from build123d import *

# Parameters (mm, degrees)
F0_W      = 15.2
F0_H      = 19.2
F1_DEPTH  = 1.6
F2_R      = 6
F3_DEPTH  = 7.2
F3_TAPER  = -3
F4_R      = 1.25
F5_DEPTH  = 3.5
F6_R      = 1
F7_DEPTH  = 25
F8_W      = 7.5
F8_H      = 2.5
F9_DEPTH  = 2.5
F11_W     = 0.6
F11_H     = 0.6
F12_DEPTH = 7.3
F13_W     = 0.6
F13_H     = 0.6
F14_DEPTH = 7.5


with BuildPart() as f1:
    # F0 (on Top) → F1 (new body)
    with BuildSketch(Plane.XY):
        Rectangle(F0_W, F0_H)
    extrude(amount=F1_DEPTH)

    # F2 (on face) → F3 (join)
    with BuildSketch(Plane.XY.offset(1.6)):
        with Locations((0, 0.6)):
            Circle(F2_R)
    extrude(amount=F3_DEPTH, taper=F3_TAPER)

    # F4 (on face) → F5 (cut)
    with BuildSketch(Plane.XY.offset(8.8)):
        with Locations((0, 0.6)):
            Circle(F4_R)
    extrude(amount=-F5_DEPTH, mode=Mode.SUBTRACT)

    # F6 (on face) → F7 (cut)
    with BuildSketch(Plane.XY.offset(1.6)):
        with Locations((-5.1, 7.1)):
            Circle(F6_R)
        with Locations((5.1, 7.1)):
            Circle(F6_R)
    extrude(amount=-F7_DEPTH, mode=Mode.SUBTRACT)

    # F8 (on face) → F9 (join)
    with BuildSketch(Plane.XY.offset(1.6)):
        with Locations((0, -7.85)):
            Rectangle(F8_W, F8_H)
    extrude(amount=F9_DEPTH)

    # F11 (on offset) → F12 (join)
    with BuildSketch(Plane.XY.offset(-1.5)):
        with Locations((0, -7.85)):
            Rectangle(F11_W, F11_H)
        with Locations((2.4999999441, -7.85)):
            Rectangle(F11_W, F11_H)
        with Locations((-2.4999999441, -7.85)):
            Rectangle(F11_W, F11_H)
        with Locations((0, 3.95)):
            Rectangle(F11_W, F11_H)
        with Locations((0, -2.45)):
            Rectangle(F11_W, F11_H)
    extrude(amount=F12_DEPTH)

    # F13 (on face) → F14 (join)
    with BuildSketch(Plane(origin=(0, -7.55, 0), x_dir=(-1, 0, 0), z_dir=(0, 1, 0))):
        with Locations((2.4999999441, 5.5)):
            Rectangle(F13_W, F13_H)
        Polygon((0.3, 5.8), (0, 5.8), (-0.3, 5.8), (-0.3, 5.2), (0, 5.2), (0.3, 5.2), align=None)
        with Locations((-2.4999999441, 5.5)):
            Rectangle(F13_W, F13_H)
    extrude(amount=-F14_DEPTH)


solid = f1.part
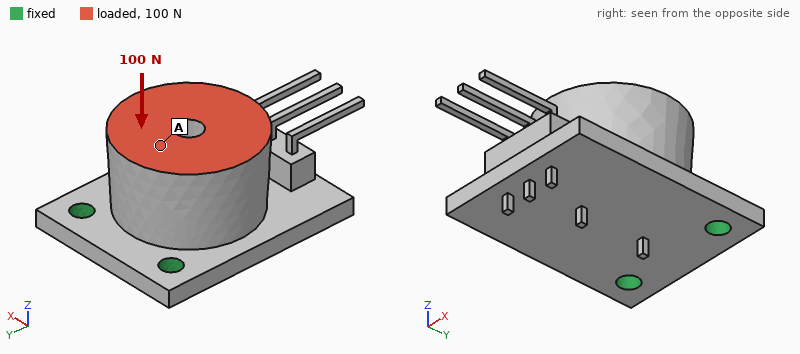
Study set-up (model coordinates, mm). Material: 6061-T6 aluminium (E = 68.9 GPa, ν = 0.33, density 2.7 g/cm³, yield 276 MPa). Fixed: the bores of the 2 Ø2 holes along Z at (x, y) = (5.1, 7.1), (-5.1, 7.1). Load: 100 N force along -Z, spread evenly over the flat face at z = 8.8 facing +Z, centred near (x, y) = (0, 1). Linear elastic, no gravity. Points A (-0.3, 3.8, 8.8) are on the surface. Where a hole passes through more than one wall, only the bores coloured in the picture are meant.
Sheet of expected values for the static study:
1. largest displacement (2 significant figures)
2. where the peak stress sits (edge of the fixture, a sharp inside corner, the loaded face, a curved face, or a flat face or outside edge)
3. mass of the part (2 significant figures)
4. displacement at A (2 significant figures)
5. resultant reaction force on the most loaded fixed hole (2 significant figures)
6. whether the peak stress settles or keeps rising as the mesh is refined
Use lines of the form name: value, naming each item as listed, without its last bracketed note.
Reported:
largest displacement: 66 µm
where the peak stress sits: edge of the fixture
mass of the part: 3.7 g
displacement at A: 25 µm
resultant reaction force on the most loaded fixed hole: 50 N
whether the peak stress settles or keeps rising as the mesh is refined: keeps rising
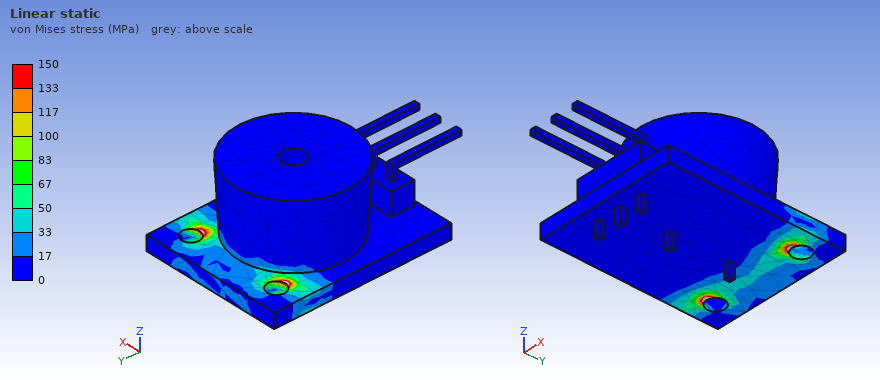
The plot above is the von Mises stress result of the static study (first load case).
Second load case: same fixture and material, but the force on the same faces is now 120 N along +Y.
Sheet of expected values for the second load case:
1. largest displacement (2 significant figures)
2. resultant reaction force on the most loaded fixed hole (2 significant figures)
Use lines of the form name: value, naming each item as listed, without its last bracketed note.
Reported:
largest displacement: 0.12 mm
resultant reaction force on the most loaded fixed hole: 63 N
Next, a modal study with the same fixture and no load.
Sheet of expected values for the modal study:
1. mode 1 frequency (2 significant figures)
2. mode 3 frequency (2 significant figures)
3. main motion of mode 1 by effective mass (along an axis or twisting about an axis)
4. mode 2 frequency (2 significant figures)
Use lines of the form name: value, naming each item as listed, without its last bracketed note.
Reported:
mode 1 frequency: 4100 Hz
mode 3 frequency: 6600 Hz
main motion of mode 1 by effective mass: along Z
mode 2 frequency: 6600 Hz
